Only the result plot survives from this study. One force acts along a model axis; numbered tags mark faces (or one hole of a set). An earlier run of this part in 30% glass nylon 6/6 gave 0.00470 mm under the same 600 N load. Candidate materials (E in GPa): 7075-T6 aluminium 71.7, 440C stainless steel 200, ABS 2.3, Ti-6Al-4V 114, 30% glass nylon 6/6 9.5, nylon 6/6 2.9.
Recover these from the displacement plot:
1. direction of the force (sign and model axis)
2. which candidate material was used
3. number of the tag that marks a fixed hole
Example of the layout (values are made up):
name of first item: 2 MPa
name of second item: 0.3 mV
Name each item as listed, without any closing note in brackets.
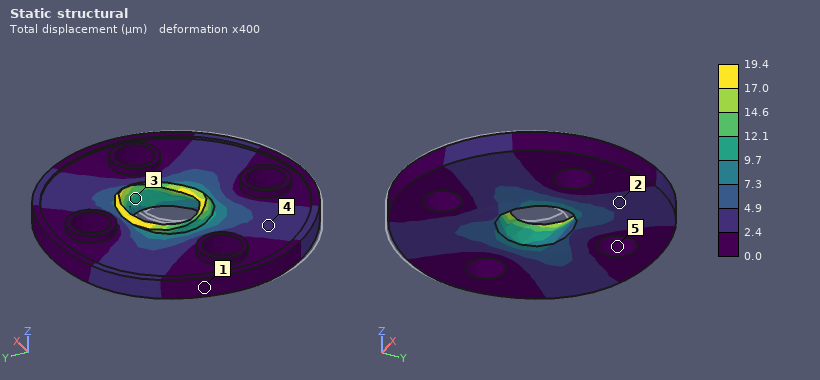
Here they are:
direction of the force: +Y
which candidate material was used: ABS
number of the tag that marks a fixed hole: 5
